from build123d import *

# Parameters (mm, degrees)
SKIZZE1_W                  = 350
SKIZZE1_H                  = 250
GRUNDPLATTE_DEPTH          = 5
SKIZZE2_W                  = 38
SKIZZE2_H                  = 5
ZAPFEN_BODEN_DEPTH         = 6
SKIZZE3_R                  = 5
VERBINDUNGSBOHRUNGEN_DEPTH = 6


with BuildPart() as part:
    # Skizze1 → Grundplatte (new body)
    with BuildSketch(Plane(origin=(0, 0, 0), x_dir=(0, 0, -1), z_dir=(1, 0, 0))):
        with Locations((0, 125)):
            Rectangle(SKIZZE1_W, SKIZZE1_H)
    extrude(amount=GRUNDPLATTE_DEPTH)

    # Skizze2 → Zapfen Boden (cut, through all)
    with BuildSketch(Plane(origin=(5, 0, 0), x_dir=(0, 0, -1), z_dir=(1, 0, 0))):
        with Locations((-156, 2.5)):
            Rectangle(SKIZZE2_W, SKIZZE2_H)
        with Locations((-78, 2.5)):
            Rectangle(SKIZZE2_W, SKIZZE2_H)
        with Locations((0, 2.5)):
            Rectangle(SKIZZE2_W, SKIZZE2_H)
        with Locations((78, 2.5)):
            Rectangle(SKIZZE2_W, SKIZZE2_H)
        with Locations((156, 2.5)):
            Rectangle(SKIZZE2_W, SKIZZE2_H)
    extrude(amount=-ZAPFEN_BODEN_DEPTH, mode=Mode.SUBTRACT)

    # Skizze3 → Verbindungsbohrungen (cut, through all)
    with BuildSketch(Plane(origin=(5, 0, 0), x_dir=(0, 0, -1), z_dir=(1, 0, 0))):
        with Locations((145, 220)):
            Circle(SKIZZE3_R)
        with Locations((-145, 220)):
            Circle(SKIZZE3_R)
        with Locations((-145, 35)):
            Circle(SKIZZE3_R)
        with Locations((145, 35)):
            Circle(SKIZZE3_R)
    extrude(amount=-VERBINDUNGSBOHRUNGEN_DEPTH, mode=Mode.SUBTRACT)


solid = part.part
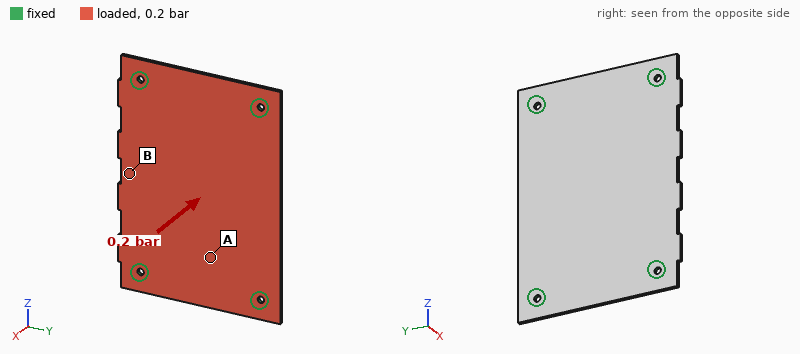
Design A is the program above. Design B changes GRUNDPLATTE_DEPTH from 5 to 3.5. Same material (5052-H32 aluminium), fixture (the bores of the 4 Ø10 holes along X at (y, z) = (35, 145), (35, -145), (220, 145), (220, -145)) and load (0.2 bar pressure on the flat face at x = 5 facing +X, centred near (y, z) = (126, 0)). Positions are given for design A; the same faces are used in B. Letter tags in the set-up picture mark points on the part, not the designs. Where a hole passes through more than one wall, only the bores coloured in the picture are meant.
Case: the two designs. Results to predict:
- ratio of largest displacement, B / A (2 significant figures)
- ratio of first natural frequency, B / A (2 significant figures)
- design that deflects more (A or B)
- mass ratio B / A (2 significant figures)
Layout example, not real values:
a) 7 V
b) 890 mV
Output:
a) 2.9
b) 0.71
c) B
d) 0.70
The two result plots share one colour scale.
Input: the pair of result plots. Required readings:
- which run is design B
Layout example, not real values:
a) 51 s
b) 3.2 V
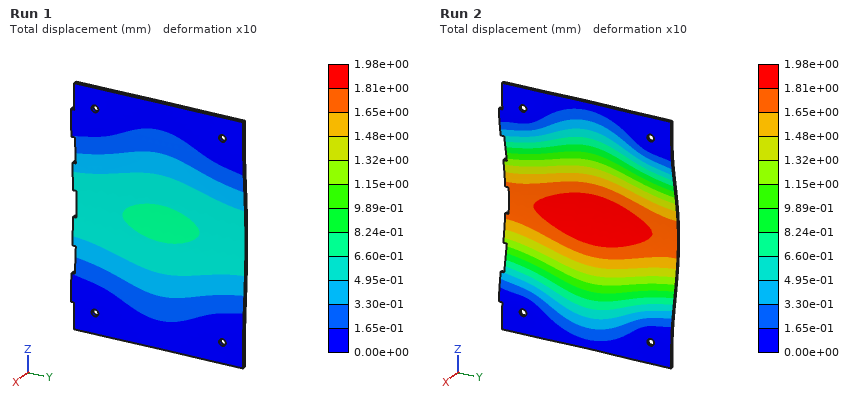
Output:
a) Run 2
